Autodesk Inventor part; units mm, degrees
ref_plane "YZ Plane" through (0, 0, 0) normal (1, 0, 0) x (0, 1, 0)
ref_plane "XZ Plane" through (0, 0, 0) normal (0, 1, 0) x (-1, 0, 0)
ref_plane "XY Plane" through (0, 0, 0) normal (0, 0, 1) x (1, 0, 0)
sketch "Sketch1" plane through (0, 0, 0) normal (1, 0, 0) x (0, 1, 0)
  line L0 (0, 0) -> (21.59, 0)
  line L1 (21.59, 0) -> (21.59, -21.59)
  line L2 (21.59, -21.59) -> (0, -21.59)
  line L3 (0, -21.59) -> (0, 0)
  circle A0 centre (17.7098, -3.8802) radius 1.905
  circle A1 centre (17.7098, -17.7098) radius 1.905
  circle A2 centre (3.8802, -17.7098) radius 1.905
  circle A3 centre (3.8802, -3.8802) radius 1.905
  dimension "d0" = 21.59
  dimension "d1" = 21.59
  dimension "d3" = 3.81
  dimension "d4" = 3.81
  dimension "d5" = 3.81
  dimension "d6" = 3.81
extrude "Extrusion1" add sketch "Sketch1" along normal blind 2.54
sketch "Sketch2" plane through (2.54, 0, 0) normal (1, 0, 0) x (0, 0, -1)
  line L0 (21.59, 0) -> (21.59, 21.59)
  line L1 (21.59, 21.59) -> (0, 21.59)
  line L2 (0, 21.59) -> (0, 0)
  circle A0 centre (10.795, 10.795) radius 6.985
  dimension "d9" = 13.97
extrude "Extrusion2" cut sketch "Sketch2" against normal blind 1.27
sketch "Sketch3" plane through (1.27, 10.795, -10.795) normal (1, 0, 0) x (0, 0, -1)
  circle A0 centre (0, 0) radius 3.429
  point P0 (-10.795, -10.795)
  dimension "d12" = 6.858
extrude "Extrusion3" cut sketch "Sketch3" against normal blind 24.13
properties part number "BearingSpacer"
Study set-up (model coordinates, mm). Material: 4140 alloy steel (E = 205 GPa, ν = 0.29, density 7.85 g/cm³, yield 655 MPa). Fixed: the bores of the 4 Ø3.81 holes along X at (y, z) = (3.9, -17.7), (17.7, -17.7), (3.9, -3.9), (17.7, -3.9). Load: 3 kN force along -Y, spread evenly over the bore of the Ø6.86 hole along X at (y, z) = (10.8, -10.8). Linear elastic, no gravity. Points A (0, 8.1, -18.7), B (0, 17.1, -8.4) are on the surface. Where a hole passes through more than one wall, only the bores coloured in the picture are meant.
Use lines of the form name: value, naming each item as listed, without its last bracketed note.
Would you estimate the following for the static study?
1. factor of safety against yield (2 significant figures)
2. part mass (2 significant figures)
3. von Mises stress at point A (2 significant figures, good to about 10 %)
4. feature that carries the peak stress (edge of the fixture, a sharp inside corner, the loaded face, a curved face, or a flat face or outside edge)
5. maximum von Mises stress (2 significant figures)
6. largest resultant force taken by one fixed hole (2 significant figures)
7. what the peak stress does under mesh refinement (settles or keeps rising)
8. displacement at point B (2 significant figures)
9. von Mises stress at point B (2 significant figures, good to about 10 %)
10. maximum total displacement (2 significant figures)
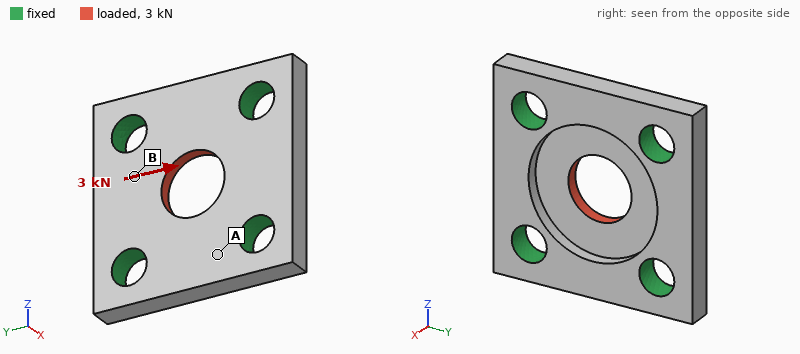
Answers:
factor of safety against yield: 3.4
part mass: 6.5 g
von Mises stress at point A: 15 MPa
feature that carries the peak stress: the loaded face
maximum von Mises stress: 190 MPa
largest resultant force taken by one fixed hole: 790 N
what the peak stress does under mesh refinement: settles
displacement at point B: 2.1 µm
von Mises stress at point B: 71 MPa
maximum total displacement: 4.0 µm
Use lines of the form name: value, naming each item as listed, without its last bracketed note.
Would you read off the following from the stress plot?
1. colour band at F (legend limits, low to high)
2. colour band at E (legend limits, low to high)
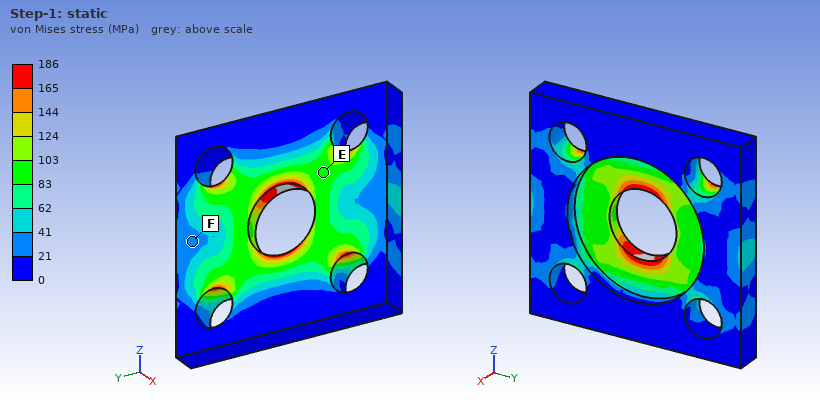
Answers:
colour band at F: 21 to 41 MPa
colour band at E: 83 to 103 MPa
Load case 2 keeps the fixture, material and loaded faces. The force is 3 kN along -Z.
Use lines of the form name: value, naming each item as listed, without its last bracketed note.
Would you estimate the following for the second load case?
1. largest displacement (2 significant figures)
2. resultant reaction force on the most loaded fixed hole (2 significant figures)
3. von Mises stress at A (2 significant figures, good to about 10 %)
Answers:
largest displacement: 4.0 µm
resultant reaction force on the most loaded fixed hole: 790 N
von Mises stress at A: 70 MPa
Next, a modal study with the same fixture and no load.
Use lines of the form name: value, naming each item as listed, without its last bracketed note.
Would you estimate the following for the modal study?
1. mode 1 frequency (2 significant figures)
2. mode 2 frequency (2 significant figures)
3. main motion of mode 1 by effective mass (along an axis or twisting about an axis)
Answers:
mode 1 frequency: 65 kHz
mode 2 frequency: 78 kHz
main motion of mode 1 by effective mass: along X
